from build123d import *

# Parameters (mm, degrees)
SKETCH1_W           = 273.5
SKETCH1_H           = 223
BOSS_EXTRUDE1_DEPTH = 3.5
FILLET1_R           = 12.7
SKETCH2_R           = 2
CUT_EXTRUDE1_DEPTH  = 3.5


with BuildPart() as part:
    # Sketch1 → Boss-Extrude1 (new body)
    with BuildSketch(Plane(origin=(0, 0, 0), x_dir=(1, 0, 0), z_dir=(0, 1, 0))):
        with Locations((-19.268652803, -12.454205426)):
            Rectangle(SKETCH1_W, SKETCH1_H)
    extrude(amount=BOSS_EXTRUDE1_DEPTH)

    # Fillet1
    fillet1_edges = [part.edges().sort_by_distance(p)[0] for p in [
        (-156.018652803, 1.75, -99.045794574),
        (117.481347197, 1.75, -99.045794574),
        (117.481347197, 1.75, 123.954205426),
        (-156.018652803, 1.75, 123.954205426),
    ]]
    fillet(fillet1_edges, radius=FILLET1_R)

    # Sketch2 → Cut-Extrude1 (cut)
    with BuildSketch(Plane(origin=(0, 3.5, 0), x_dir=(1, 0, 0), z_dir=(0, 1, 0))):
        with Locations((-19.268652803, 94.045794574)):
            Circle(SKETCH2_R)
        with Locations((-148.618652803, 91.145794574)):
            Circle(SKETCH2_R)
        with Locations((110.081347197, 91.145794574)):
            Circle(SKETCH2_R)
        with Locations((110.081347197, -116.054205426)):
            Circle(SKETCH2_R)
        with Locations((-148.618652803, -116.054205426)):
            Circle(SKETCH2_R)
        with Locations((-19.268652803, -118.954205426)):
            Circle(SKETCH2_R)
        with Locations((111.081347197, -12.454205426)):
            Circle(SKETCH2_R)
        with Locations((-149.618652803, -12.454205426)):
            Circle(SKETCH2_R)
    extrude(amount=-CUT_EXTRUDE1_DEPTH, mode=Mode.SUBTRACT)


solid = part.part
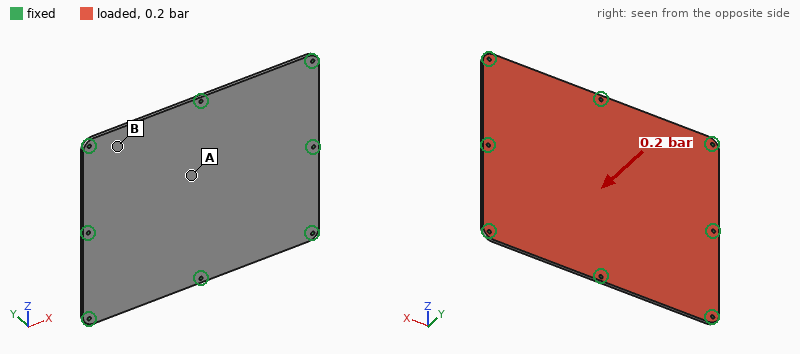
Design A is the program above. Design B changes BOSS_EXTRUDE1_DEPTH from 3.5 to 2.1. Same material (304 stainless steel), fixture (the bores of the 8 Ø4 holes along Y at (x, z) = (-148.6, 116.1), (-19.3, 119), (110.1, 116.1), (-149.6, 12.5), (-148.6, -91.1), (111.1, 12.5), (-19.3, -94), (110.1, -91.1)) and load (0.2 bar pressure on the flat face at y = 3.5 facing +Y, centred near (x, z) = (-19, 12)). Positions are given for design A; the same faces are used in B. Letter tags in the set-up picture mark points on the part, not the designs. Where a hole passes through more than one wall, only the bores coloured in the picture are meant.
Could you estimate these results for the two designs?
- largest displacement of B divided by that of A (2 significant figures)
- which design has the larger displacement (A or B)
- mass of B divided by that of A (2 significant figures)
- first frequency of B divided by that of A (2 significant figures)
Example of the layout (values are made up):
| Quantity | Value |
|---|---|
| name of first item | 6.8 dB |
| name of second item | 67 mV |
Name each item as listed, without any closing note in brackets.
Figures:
| Quantity | Value |
|---|---|
| largest displacement of B divided by that of A | 4.5 |
| which design has the larger displacement | B |
| mass of B divided by that of A | 0.60 |
| first frequency of B divided by that of A | 0.61 |
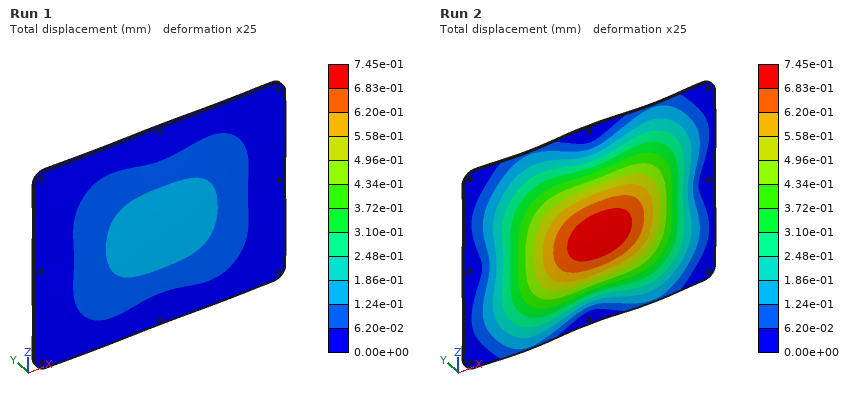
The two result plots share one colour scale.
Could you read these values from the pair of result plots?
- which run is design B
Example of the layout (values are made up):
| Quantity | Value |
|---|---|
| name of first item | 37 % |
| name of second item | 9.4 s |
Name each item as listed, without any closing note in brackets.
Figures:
| Quantity | Value |
|---|---|
| which run is design B | Run 2 |
